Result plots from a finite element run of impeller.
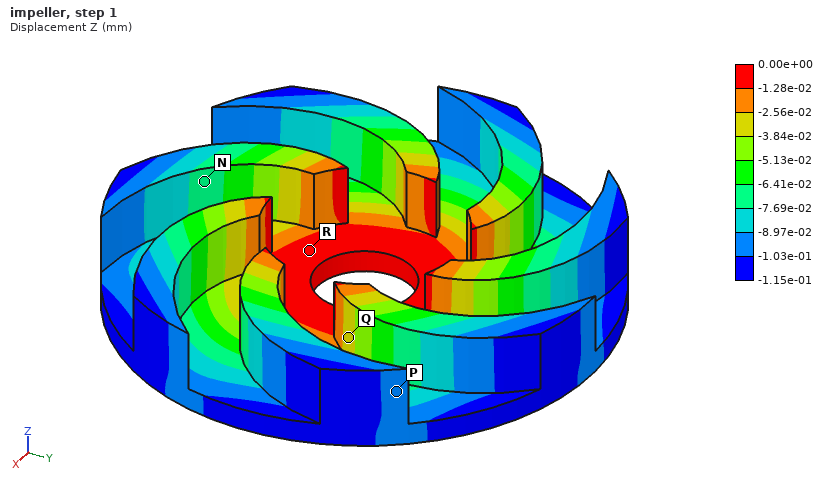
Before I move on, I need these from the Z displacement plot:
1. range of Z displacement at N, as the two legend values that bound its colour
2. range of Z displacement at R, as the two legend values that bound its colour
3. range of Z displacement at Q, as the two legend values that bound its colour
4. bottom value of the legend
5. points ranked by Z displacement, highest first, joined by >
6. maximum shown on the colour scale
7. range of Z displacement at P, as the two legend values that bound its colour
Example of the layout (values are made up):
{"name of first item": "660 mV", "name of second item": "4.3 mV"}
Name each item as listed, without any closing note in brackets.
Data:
{"range of Z displacement at N, as the two legend values that bound its colour": "-7.69e-02 to -6.41e-02 mm", "range of Z displacement at R, as the two legend values that bound its colour": "-1.28e-02 to 0.00e+00 mm", "range of Z displacement at Q, as the two legend values that bound its colour": "-3.84e-02 to -2.56e-02 mm", "bottom value of the legend": "-1.15e-01 mm", "points ranked by Z displacement, highest first, joined by >": "R > Q > N > P", "maximum shown on the colour scale": "0.00e+00 mm", "range of Z displacement at P, as the two legend values that bound its colour": "-1.03e-01 to -8.97e-02 mm"}
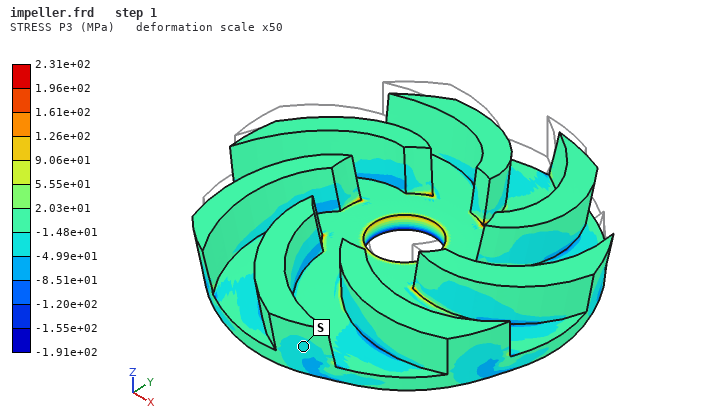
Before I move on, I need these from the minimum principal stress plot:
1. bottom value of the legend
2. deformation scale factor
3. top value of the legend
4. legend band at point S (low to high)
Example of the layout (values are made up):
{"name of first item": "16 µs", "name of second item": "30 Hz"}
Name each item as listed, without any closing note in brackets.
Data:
{"bottom value of the legend": "-1.91e+02 MPa", "deformation scale factor": "50", "top value of the legend": "2.31e+02 MPa", "legend band at point S": "-4.99e+01 to -1.48e+01 MPa"}
